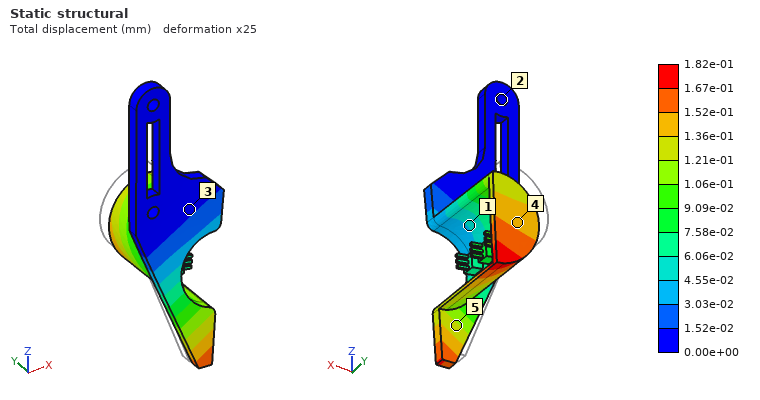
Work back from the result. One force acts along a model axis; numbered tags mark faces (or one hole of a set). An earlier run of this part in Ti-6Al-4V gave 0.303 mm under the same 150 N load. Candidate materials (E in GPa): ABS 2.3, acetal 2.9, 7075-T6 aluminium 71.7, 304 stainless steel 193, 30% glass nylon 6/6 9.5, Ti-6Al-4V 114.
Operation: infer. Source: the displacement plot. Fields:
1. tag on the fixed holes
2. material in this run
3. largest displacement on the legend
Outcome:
2
304 stainless steel
1.82e-01 mm
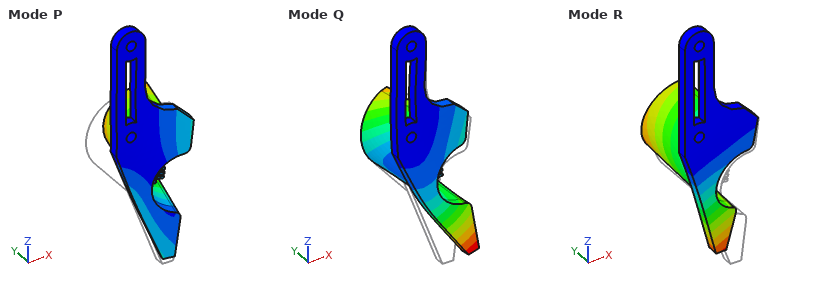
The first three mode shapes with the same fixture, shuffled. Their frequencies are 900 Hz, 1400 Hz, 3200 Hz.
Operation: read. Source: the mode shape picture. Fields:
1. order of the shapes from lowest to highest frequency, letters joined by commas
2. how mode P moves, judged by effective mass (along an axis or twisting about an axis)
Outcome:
R, P, Q
along X
